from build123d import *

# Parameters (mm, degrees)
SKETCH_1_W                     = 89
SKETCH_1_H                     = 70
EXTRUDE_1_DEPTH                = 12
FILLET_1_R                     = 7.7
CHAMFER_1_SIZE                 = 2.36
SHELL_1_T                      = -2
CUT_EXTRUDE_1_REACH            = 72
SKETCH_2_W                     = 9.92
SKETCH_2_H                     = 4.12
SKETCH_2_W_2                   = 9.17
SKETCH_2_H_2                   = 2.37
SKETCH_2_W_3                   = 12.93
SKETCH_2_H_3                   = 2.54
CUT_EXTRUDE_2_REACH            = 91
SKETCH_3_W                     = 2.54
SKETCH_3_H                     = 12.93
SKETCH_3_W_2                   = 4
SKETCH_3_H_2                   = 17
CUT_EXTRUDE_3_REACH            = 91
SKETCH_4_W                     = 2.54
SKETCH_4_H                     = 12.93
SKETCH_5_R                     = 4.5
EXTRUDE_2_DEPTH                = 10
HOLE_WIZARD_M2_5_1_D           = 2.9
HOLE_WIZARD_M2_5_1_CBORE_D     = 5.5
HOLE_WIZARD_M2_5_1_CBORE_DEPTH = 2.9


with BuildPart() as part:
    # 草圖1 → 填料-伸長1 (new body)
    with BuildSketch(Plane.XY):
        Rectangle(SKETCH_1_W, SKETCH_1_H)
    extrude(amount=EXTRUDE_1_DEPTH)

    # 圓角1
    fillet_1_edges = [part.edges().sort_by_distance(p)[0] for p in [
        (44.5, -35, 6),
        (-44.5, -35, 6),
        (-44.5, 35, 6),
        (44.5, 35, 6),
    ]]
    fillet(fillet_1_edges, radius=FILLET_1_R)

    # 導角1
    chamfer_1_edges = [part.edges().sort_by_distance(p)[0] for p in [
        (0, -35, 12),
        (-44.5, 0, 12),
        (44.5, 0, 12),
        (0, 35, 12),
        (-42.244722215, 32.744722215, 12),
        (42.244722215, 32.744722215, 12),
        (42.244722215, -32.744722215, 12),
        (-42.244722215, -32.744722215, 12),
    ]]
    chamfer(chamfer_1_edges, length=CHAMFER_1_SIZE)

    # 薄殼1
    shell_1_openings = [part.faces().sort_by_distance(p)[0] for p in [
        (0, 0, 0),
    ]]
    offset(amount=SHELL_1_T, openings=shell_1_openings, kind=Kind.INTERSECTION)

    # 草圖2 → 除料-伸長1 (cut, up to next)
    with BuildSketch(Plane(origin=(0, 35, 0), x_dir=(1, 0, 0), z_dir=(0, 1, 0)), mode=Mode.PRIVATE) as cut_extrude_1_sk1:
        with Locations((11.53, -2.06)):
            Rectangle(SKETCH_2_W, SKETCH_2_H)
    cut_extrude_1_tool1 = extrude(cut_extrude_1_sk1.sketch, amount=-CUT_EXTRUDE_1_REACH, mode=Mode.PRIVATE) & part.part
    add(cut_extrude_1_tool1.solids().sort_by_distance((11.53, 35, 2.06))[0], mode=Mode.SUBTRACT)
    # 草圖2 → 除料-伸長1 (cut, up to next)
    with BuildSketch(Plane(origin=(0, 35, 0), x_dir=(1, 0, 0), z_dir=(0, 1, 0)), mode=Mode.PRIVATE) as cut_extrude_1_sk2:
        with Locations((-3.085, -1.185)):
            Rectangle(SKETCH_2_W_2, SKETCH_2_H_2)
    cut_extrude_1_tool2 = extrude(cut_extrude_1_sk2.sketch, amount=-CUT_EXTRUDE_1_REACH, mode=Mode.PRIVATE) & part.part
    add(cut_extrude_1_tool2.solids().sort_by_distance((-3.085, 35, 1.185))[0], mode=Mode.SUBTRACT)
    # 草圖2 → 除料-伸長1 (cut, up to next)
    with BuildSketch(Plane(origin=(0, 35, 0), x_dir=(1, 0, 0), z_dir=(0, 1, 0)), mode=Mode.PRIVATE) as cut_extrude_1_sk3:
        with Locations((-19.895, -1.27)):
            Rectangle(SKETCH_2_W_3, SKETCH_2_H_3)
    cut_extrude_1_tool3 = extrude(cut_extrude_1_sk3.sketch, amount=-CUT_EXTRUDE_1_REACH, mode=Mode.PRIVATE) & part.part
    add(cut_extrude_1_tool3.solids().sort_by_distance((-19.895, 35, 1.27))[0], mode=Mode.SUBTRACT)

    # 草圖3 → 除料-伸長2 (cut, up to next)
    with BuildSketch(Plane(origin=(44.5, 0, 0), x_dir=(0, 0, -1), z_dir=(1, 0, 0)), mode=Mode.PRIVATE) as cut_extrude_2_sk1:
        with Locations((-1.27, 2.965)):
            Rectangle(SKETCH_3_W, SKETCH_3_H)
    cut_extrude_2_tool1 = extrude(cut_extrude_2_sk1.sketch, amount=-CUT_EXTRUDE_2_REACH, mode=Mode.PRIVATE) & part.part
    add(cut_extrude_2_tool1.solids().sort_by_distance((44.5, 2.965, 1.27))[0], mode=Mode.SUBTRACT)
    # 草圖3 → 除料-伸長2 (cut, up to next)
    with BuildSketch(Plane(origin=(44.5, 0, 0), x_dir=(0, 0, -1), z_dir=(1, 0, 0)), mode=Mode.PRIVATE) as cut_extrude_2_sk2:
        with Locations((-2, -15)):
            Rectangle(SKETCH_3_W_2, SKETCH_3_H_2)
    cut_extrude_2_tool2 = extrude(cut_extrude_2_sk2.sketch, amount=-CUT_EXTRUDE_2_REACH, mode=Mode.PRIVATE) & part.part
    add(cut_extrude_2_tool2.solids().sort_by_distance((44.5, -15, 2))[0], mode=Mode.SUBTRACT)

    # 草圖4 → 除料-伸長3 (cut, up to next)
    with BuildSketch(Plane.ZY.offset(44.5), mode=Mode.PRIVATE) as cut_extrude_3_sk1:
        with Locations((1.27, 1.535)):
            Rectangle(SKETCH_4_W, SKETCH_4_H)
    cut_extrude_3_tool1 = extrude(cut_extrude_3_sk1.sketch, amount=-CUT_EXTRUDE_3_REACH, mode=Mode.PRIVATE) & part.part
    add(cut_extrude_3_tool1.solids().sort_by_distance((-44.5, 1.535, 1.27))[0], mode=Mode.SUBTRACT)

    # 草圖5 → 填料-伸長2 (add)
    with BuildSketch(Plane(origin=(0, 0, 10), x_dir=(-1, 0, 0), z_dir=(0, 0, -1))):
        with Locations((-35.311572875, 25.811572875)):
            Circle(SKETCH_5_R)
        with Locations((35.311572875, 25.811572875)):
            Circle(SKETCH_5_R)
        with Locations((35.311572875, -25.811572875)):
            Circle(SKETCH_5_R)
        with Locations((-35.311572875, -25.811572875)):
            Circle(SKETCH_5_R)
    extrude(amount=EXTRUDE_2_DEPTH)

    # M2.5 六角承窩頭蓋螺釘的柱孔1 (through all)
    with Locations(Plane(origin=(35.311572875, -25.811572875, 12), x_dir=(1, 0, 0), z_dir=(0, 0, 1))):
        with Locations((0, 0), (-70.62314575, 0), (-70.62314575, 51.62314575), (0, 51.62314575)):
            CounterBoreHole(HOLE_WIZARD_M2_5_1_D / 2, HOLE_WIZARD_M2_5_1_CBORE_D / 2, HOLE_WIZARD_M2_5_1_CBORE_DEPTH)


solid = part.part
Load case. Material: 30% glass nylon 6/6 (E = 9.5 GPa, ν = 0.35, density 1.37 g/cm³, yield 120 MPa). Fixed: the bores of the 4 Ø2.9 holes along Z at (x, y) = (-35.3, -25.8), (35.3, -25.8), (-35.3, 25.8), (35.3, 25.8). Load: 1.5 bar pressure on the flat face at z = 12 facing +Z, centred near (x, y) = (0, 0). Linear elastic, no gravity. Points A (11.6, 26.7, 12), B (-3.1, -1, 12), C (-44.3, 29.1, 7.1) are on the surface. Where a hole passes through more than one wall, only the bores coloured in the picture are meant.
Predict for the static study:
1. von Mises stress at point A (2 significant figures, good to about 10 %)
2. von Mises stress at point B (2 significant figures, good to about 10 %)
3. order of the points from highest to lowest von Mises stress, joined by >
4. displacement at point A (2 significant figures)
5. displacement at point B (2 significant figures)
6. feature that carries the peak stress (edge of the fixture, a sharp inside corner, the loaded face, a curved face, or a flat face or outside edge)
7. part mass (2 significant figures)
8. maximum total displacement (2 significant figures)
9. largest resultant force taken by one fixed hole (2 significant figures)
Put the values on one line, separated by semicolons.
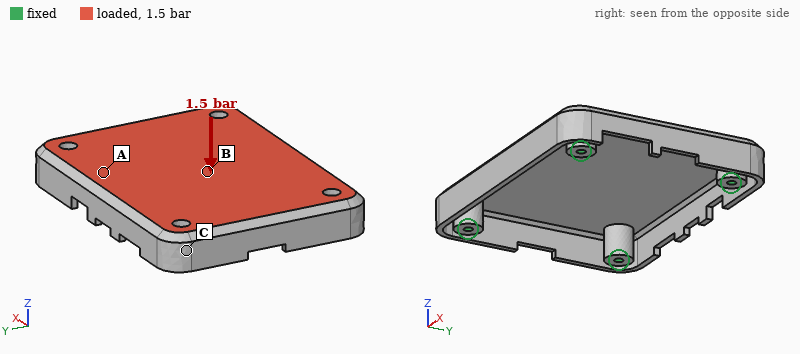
21 MPa; 40 MPa; B > A > C; 0.45 mm; 1.3 mm; the loaded face; 26 g; 1.3 mm; 250 N
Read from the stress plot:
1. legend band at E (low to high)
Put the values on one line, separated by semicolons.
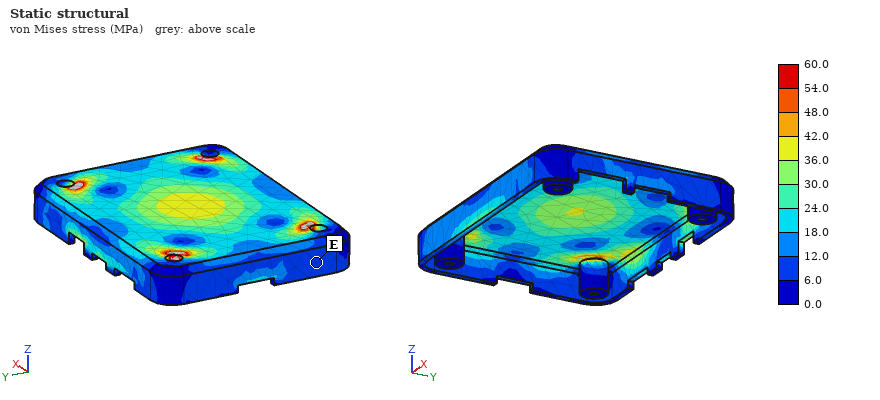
6.0 to 12.0 MPa
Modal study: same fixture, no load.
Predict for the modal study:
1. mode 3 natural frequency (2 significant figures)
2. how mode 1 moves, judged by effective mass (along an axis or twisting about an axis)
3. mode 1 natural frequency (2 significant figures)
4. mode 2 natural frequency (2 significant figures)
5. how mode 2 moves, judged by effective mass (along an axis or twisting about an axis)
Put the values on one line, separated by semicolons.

2600 Hz; along Z; 1300 Hz; 2300 Hz; twisting about X
